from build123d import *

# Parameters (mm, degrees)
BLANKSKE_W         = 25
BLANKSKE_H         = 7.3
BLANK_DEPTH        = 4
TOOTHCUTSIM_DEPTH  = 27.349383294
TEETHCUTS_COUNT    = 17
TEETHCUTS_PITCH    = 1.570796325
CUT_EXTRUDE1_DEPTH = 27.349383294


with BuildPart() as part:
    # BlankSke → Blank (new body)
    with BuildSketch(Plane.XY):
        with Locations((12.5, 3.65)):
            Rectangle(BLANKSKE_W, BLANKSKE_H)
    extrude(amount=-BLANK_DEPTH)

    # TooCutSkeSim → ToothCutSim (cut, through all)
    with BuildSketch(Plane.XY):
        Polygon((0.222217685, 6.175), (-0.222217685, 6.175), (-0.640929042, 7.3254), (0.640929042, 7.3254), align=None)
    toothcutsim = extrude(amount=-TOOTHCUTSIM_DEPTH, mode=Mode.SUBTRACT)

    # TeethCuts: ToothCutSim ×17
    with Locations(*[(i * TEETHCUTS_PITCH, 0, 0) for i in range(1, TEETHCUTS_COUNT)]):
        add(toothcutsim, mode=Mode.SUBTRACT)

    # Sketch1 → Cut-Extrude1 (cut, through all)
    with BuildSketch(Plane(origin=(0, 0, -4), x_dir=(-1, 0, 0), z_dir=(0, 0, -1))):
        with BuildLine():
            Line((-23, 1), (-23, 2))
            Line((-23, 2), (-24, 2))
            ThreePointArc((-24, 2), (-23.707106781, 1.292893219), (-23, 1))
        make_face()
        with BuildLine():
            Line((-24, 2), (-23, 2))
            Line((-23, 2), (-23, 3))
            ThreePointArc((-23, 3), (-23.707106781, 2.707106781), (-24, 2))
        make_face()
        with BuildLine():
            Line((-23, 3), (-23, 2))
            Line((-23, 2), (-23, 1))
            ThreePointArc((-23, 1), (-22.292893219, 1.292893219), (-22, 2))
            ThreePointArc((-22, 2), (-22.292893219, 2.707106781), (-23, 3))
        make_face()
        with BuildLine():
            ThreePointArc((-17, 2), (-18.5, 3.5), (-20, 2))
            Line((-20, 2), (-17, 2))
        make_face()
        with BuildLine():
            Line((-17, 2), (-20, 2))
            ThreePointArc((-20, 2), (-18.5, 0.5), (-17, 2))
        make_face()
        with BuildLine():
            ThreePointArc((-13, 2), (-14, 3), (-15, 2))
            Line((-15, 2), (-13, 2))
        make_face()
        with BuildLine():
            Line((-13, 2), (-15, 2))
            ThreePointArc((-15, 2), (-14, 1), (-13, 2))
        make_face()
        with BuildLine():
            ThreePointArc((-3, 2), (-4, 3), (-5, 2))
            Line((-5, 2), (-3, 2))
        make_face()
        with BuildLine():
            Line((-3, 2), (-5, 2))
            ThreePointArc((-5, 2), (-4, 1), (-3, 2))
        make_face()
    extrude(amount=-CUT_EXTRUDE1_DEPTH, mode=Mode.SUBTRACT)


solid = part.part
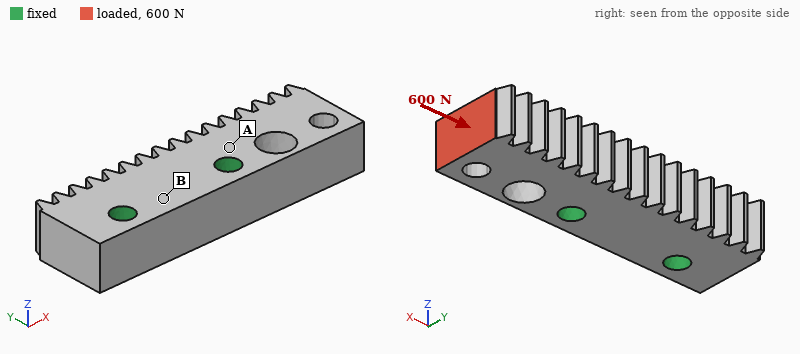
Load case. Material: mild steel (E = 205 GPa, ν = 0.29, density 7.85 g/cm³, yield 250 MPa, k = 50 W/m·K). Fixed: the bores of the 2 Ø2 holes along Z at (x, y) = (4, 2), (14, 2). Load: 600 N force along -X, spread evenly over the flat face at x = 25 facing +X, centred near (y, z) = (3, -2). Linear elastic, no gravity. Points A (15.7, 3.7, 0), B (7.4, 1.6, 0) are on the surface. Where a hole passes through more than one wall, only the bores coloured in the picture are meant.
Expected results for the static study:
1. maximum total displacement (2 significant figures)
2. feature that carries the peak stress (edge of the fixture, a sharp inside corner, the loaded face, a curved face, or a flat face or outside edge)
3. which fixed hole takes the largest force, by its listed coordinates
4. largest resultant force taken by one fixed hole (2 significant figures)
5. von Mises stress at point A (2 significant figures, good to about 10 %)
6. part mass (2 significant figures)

3.0 µm
a curved face
(14, 2)
520 N
34 MPa
4.7 g
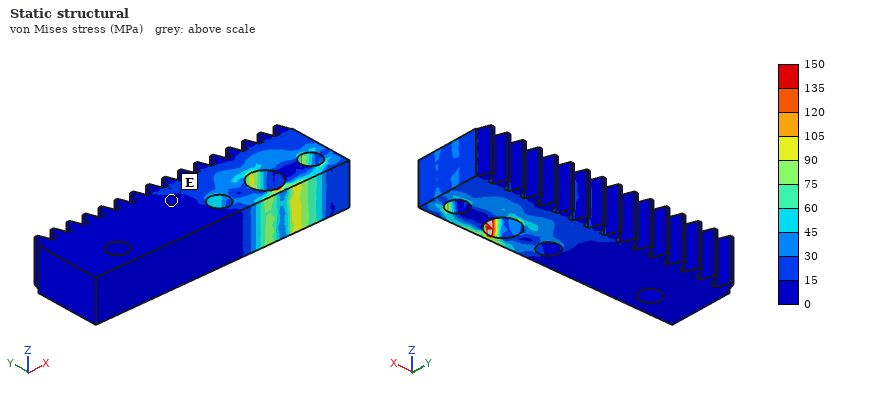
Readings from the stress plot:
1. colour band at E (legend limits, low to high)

0 to 15 MPa
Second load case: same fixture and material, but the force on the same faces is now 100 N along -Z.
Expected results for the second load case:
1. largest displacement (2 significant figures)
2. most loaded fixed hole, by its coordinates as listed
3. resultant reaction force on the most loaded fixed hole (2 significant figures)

11 µm
(14, 2)
120 N
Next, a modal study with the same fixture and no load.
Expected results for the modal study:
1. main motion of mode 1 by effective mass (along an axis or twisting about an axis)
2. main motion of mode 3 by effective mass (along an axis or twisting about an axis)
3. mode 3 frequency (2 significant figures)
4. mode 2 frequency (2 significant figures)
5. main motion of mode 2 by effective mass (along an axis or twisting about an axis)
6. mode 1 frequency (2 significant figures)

along Z
twisting about X
49 kHz
26 kHz
along Y
22 kHz
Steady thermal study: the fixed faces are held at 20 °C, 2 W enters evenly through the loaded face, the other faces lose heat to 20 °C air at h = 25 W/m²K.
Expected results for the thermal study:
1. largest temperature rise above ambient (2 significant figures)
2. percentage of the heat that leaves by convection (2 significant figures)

24 K
4.9 %
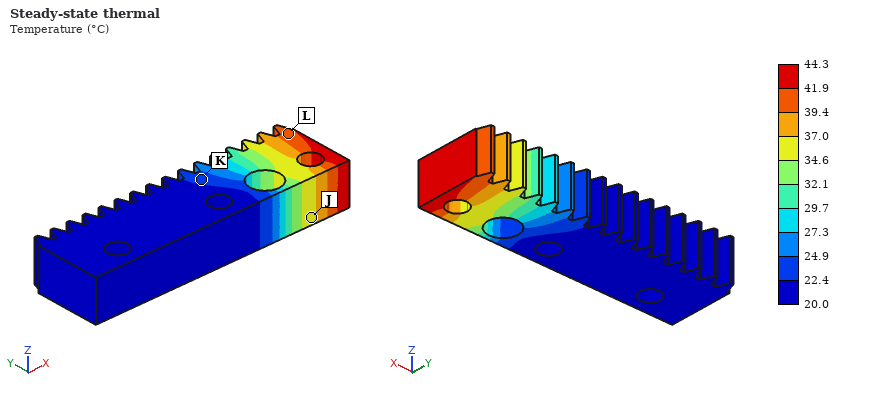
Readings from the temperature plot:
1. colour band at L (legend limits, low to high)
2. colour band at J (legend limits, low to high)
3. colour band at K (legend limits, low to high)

39.4 to 41.9 °C
34.6 to 37.0 °C
22.4 to 24.9 °C
